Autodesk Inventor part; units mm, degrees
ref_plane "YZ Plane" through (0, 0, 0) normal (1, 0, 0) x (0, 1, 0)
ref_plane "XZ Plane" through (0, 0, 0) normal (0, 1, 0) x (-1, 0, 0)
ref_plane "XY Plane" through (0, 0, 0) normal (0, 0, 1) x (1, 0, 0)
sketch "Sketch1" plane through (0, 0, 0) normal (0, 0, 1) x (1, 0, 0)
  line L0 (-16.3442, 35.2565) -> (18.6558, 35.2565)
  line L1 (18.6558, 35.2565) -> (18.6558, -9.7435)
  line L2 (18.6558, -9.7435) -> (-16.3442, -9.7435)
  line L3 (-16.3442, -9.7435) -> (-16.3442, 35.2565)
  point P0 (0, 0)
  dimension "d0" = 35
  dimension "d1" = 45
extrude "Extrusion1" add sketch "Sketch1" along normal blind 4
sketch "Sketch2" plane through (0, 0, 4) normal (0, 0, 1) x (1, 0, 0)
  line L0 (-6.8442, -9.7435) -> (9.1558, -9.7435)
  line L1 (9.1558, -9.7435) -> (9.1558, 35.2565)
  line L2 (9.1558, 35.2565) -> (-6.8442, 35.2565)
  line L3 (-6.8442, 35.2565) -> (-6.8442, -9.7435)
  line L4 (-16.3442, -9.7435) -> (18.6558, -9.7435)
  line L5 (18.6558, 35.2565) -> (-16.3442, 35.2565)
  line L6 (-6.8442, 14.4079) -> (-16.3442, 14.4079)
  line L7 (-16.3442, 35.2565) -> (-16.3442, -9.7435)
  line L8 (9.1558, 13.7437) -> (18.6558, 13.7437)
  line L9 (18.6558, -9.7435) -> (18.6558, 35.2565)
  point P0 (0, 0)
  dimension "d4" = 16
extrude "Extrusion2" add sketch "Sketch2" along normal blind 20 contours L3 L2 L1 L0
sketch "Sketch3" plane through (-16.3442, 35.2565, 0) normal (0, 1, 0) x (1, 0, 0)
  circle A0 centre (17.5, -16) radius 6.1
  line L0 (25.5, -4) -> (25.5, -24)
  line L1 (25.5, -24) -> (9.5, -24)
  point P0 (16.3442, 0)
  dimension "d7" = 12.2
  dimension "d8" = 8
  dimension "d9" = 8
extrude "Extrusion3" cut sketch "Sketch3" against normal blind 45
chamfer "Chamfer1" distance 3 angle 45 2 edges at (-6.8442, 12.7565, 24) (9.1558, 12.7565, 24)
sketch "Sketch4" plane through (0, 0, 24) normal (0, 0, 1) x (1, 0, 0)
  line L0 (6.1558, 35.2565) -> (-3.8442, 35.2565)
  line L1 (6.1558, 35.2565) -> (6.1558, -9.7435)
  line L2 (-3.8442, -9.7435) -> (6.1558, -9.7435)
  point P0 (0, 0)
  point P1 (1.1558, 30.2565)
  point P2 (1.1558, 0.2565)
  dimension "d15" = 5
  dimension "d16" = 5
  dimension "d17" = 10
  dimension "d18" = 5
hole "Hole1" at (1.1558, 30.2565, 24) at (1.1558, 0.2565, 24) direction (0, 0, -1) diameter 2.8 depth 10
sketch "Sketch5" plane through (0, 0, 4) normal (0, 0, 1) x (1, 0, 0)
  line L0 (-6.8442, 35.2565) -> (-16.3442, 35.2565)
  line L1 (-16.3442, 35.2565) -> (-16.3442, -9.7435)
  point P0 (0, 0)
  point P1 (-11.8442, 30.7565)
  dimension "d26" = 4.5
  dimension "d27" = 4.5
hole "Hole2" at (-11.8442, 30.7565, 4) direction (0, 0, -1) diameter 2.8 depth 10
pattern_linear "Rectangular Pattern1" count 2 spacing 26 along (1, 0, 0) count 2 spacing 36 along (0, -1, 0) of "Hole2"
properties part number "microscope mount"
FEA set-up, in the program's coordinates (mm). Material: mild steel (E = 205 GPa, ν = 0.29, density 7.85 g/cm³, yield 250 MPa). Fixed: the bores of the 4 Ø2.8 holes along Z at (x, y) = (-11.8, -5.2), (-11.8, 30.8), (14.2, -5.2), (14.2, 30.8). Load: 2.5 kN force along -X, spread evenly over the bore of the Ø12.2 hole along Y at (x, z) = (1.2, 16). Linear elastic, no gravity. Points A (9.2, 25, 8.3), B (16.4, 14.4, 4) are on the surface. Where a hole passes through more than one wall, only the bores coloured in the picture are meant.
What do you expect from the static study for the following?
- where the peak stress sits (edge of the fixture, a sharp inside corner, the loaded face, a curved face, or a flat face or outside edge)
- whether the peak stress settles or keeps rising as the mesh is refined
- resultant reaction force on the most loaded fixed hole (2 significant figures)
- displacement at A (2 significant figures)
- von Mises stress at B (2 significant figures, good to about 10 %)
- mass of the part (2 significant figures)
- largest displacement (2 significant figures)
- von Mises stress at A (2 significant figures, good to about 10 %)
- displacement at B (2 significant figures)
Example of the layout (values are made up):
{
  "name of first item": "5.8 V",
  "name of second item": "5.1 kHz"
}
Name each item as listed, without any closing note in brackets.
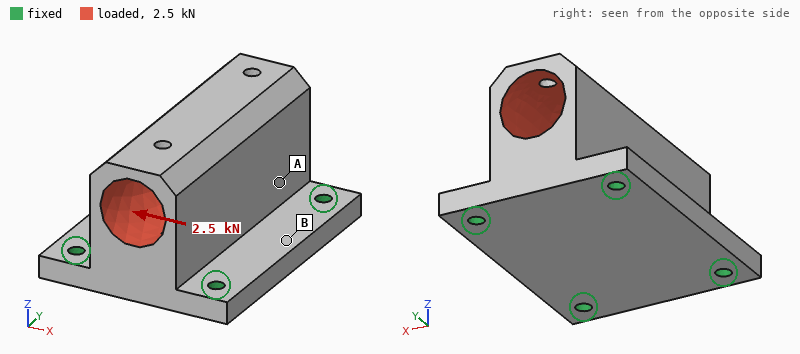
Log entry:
{
  "where the peak stress sits": "edge of the fixture",
  "whether the peak stress settles or keeps rising as the mesh is refined": "keeps rising",
  "resultant reaction force on the most loaded fixed hole": "1.0 kN",
  "displacement at A": "4.2 µm",
  "von Mises stress at B": "13 MPa",
  "mass of the part": "120 g",
  "largest displacement": "15 µm",
  "von Mises stress at A": "27 MPa",
  "displacement at B": "4.3 µm"
}
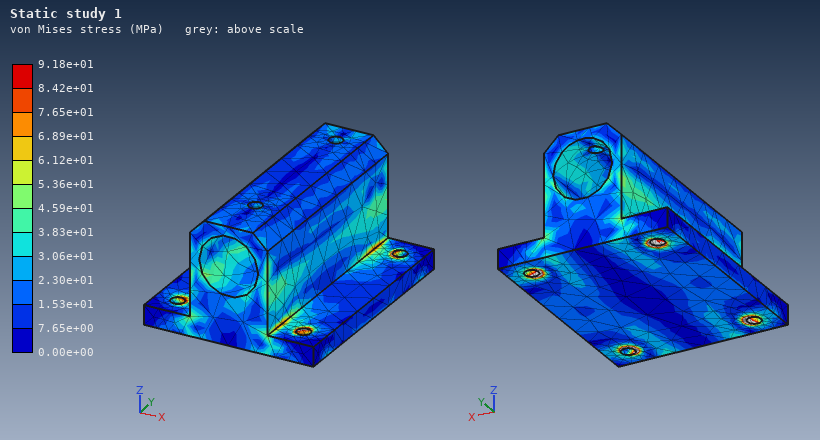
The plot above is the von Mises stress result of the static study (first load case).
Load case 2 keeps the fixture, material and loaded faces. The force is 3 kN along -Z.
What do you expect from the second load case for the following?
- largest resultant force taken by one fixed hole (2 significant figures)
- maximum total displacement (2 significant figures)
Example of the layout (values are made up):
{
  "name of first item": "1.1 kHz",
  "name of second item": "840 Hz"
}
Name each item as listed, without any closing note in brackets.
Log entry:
{
  "largest resultant force taken by one fixed hole": "800 N",
  "maximum total displacement": "5.4 µm"
}
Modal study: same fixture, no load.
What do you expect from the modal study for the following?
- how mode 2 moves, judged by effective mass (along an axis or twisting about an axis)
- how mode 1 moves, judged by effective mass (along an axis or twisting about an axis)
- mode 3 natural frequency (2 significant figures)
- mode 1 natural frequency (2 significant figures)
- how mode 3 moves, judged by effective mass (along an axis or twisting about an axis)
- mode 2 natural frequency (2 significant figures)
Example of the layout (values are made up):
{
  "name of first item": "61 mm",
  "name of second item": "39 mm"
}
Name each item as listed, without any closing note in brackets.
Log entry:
{
  "how mode 2 moves, judged by effective mass": "along Z",
  "how mode 1 moves, judged by effective mass": "along X",
  "mode 3 natural frequency": "15 kHz",
  "mode 1 natural frequency": "11 kHz",
  "how mode 3 moves, judged by effective mass": "along Y",
  "mode 2 natural frequency": "14 kHz"
}
